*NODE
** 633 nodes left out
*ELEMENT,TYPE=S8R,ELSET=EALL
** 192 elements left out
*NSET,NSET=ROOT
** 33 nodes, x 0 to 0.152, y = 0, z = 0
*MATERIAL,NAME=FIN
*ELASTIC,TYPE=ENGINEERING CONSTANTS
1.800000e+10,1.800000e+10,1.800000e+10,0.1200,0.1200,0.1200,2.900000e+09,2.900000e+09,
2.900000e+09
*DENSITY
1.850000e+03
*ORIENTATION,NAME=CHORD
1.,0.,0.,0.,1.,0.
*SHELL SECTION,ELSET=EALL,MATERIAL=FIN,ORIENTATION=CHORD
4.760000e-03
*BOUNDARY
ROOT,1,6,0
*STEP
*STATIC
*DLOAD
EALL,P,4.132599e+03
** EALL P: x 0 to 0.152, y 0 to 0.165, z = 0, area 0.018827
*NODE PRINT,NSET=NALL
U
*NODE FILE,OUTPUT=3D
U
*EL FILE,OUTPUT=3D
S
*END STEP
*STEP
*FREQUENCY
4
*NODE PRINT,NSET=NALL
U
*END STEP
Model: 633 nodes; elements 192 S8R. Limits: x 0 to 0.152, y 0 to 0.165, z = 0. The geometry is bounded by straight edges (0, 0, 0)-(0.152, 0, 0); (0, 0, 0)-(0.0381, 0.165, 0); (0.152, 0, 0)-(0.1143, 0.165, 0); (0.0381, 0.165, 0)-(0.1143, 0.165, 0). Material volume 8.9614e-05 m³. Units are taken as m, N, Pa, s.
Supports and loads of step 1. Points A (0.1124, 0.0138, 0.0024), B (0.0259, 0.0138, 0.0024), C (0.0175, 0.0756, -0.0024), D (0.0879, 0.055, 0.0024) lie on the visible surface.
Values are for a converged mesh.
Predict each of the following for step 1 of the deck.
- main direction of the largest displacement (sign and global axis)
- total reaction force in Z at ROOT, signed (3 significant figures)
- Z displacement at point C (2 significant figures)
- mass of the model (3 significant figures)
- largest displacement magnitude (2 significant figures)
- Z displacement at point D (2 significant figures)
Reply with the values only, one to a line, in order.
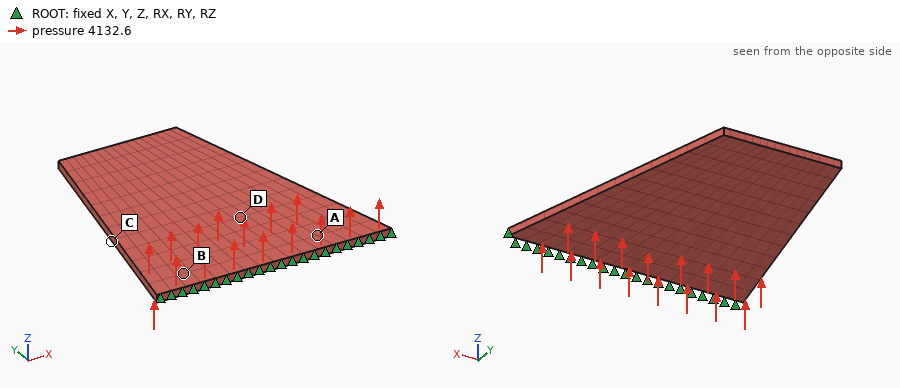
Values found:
+Z
-77.8 N
4.9e-04 m
0.166 kg
0.0017 m
3.0e-04 m
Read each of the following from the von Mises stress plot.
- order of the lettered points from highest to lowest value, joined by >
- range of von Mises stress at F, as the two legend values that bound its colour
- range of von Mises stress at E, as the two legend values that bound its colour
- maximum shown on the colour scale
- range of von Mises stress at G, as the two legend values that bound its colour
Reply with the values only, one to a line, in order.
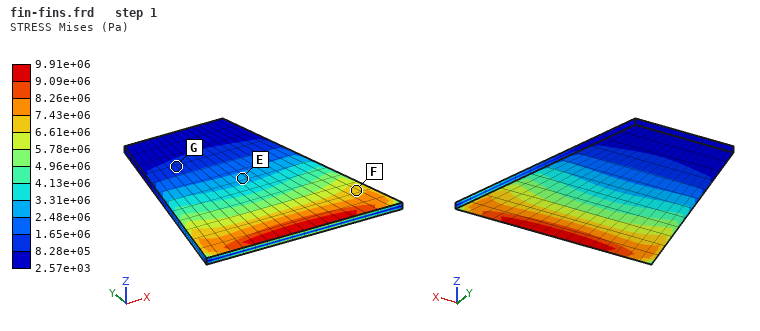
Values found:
F > E > G
6.61e+06 to 7.43e+06 Pa
2.48e+06 to 3.31e+06 Pa
9.91e+06 Pa
8.28e+05 to 1.65e+06 Pa
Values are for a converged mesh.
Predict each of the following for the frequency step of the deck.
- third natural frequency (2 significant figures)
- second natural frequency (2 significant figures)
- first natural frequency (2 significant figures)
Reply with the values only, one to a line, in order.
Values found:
580 Hz
300 Hz
110 Hz
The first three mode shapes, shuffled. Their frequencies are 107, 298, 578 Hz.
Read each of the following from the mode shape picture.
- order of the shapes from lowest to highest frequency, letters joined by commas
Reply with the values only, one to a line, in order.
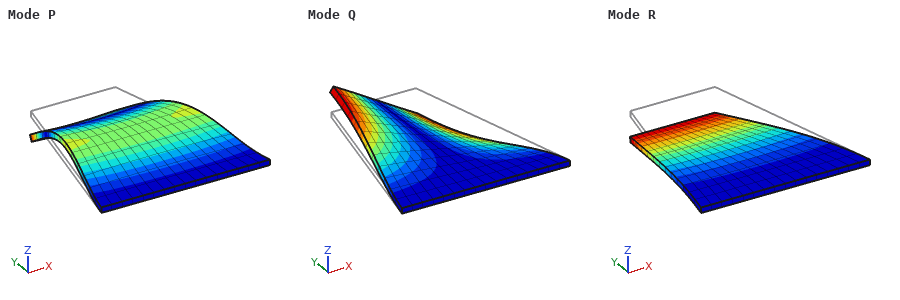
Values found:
R, Q, P
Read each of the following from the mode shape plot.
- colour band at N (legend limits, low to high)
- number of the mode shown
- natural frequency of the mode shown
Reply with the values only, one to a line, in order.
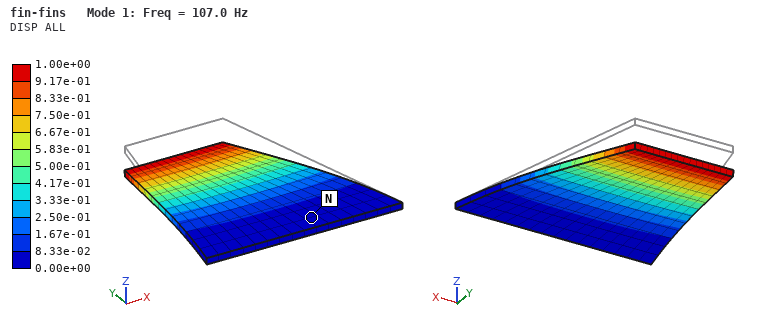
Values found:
0.00e+00 to 8.33e-02
1
107.0 Hz
